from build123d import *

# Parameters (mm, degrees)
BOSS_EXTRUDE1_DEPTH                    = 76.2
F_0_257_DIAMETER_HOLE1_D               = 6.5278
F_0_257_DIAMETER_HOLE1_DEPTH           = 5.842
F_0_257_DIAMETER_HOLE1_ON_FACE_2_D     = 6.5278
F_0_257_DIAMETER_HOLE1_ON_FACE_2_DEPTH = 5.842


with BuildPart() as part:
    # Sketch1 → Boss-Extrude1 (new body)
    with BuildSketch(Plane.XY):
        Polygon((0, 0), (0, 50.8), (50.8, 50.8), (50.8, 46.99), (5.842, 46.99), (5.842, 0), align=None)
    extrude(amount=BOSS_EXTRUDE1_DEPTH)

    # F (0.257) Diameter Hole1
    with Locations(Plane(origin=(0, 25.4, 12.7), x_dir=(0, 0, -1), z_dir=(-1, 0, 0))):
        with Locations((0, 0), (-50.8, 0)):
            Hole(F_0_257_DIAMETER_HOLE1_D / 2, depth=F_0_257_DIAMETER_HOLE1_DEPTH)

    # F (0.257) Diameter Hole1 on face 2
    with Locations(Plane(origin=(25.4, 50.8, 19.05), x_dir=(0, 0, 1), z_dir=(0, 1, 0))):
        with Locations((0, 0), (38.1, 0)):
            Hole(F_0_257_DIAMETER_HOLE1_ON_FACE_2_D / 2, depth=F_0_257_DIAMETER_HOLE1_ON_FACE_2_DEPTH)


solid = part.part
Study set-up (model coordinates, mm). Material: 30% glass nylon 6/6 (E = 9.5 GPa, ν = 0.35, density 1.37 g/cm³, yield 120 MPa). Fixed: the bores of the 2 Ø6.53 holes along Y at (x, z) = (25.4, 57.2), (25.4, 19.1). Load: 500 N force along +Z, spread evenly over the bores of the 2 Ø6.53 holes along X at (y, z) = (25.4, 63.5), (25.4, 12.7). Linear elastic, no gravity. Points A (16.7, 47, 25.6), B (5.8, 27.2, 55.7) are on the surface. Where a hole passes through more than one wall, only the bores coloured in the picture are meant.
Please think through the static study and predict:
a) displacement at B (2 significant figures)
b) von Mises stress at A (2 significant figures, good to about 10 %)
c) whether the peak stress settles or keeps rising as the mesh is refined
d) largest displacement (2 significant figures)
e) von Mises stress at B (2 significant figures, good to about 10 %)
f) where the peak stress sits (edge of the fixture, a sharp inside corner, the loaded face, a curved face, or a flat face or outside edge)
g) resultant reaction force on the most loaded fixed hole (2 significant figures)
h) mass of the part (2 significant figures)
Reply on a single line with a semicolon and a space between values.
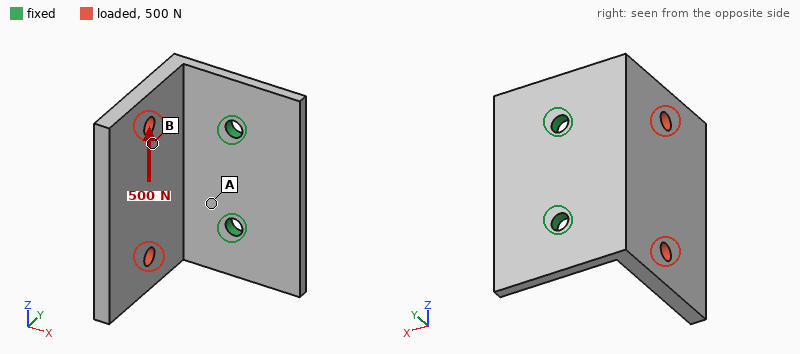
0.31 mm; 20 MPa; keeps rising; 0.68 mm; 7.0 MPa; edge of the fixture; 440 N; 48 g
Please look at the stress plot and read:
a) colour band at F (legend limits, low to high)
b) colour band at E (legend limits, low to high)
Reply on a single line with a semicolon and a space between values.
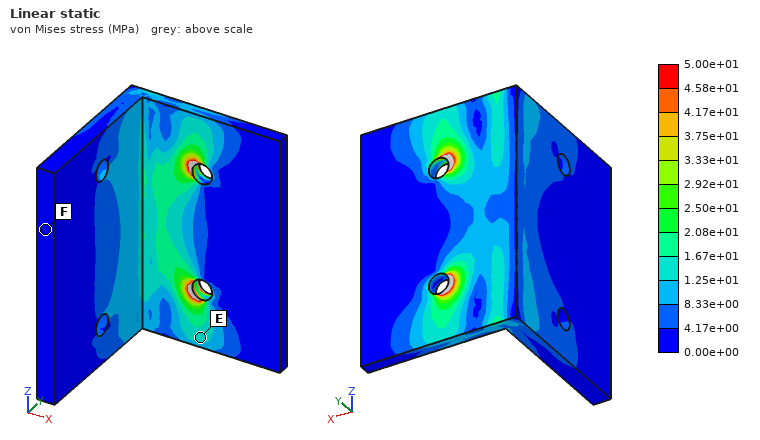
0.00e+00 to 4.17e+00 MPa; 1.25e+01 to 1.67e+01 MPa
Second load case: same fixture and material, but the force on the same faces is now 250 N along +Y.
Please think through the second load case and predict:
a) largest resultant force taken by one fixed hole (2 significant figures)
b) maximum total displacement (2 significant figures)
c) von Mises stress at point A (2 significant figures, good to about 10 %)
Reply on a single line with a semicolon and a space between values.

130 N; 0.92 mm; 18 MPa
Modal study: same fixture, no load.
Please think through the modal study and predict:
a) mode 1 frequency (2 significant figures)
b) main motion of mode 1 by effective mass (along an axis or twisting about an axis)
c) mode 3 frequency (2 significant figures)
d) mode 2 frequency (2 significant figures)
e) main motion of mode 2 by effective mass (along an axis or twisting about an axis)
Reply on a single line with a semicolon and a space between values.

370 Hz; along X; 1500 Hz; 830 Hz; along Z
